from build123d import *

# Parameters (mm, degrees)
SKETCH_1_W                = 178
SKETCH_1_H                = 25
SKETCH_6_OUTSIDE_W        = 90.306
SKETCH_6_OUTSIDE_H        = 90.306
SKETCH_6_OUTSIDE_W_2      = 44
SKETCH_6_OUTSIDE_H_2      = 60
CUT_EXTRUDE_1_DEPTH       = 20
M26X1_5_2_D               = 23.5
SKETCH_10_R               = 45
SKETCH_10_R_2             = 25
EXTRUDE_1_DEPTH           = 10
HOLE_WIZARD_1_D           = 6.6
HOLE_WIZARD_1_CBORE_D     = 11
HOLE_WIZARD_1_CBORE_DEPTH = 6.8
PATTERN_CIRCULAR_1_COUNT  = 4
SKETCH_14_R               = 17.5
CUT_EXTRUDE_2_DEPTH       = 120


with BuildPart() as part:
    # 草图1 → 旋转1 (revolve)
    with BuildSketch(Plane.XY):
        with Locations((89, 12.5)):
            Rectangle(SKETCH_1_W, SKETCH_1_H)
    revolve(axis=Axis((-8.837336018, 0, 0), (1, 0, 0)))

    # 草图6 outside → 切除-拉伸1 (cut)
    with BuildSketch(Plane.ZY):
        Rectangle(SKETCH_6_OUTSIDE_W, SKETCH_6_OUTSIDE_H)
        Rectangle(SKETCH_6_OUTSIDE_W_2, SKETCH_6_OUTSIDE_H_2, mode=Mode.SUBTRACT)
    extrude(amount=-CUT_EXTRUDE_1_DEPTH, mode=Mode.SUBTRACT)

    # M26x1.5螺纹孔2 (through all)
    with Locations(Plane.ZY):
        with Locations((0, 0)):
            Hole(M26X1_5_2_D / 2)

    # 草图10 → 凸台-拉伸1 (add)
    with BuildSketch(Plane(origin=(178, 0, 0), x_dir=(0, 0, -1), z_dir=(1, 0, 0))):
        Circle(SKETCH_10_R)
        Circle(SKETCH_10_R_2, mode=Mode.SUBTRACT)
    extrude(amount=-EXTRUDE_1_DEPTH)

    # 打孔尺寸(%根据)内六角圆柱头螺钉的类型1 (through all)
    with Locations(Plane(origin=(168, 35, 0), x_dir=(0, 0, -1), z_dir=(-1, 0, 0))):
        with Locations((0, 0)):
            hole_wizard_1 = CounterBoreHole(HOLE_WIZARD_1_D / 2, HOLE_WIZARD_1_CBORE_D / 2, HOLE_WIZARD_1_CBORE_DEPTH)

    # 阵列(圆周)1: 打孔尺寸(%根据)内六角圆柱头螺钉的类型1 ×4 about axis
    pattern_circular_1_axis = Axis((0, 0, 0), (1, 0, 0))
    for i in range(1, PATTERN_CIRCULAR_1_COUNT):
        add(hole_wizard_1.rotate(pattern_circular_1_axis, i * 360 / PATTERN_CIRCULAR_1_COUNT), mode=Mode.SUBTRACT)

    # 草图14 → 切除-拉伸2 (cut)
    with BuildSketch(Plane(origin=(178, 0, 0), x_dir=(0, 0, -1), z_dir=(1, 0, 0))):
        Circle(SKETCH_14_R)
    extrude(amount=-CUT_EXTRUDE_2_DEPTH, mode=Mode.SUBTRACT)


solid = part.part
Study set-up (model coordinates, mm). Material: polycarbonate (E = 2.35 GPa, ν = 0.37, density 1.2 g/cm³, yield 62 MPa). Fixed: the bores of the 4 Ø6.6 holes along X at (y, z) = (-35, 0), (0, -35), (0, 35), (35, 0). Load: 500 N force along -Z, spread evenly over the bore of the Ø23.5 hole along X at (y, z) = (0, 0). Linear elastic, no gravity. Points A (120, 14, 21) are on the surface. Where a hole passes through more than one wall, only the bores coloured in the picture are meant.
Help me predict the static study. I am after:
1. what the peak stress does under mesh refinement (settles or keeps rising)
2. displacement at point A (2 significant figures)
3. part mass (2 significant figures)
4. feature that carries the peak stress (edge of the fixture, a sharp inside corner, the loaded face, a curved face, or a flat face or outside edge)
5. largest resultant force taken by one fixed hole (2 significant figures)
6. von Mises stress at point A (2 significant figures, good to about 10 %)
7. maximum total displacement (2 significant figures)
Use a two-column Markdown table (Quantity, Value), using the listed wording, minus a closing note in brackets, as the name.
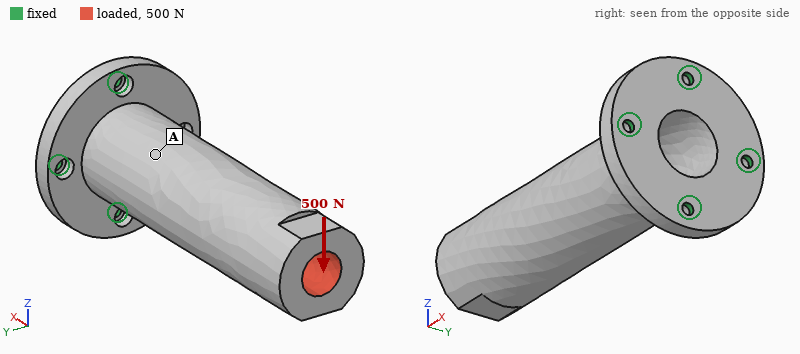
| Quantity | Value |
|---|---|
| what the peak stress does under mesh refinement | keeps rising |
| displacement at point A | 0.62 mm |
| part mass | 300 g |
| feature that carries the peak stress | edge of the fixture |
| largest resultant force taken by one fixed hole | 1.2 kN |
| von Mises stress at point A | 4.1 MPa |
| maximum total displacement | 2.5 mm |
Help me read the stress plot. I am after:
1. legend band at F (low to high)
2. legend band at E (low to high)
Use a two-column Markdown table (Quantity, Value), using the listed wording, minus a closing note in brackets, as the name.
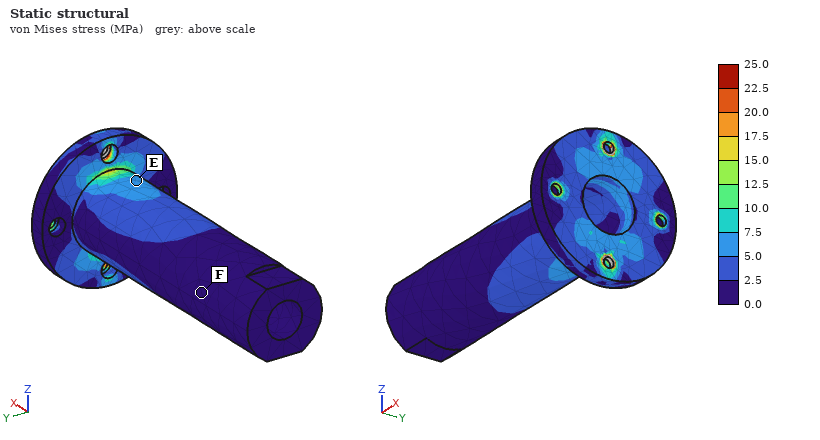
| Quantity | Value |
|---|---|
| legend band at F | 0.0 to 2.5 MPa |
| legend band at E | 5.0 to 7.5 MPa |
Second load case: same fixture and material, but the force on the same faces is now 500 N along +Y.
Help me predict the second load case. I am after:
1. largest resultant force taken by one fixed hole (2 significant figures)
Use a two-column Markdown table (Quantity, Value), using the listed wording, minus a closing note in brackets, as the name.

| Quantity | Value |
|---|---|
| largest resultant force taken by one fixed hole | 1.2 kN |
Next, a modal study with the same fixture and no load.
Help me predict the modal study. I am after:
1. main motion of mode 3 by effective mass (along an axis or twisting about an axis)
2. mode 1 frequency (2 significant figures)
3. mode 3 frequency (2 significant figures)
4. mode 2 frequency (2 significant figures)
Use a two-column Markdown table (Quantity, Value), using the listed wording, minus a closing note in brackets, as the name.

| Quantity | Value |
|---|---|
| main motion of mode 3 by effective mass | twisting about X |
| mode 1 frequency | 220 Hz |
| mode 3 frequency | 1100 Hz |
| mode 2 frequency | 220 Hz |
